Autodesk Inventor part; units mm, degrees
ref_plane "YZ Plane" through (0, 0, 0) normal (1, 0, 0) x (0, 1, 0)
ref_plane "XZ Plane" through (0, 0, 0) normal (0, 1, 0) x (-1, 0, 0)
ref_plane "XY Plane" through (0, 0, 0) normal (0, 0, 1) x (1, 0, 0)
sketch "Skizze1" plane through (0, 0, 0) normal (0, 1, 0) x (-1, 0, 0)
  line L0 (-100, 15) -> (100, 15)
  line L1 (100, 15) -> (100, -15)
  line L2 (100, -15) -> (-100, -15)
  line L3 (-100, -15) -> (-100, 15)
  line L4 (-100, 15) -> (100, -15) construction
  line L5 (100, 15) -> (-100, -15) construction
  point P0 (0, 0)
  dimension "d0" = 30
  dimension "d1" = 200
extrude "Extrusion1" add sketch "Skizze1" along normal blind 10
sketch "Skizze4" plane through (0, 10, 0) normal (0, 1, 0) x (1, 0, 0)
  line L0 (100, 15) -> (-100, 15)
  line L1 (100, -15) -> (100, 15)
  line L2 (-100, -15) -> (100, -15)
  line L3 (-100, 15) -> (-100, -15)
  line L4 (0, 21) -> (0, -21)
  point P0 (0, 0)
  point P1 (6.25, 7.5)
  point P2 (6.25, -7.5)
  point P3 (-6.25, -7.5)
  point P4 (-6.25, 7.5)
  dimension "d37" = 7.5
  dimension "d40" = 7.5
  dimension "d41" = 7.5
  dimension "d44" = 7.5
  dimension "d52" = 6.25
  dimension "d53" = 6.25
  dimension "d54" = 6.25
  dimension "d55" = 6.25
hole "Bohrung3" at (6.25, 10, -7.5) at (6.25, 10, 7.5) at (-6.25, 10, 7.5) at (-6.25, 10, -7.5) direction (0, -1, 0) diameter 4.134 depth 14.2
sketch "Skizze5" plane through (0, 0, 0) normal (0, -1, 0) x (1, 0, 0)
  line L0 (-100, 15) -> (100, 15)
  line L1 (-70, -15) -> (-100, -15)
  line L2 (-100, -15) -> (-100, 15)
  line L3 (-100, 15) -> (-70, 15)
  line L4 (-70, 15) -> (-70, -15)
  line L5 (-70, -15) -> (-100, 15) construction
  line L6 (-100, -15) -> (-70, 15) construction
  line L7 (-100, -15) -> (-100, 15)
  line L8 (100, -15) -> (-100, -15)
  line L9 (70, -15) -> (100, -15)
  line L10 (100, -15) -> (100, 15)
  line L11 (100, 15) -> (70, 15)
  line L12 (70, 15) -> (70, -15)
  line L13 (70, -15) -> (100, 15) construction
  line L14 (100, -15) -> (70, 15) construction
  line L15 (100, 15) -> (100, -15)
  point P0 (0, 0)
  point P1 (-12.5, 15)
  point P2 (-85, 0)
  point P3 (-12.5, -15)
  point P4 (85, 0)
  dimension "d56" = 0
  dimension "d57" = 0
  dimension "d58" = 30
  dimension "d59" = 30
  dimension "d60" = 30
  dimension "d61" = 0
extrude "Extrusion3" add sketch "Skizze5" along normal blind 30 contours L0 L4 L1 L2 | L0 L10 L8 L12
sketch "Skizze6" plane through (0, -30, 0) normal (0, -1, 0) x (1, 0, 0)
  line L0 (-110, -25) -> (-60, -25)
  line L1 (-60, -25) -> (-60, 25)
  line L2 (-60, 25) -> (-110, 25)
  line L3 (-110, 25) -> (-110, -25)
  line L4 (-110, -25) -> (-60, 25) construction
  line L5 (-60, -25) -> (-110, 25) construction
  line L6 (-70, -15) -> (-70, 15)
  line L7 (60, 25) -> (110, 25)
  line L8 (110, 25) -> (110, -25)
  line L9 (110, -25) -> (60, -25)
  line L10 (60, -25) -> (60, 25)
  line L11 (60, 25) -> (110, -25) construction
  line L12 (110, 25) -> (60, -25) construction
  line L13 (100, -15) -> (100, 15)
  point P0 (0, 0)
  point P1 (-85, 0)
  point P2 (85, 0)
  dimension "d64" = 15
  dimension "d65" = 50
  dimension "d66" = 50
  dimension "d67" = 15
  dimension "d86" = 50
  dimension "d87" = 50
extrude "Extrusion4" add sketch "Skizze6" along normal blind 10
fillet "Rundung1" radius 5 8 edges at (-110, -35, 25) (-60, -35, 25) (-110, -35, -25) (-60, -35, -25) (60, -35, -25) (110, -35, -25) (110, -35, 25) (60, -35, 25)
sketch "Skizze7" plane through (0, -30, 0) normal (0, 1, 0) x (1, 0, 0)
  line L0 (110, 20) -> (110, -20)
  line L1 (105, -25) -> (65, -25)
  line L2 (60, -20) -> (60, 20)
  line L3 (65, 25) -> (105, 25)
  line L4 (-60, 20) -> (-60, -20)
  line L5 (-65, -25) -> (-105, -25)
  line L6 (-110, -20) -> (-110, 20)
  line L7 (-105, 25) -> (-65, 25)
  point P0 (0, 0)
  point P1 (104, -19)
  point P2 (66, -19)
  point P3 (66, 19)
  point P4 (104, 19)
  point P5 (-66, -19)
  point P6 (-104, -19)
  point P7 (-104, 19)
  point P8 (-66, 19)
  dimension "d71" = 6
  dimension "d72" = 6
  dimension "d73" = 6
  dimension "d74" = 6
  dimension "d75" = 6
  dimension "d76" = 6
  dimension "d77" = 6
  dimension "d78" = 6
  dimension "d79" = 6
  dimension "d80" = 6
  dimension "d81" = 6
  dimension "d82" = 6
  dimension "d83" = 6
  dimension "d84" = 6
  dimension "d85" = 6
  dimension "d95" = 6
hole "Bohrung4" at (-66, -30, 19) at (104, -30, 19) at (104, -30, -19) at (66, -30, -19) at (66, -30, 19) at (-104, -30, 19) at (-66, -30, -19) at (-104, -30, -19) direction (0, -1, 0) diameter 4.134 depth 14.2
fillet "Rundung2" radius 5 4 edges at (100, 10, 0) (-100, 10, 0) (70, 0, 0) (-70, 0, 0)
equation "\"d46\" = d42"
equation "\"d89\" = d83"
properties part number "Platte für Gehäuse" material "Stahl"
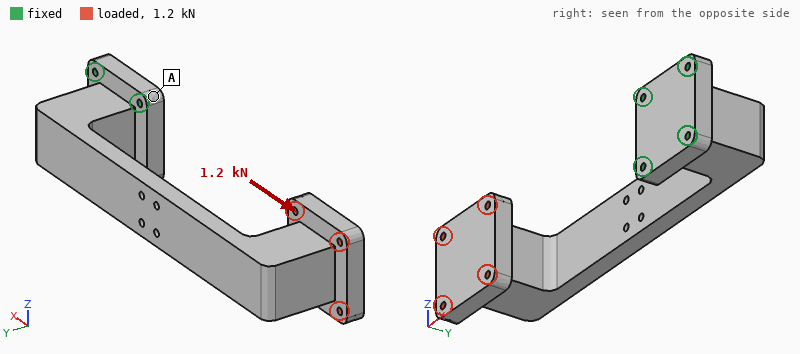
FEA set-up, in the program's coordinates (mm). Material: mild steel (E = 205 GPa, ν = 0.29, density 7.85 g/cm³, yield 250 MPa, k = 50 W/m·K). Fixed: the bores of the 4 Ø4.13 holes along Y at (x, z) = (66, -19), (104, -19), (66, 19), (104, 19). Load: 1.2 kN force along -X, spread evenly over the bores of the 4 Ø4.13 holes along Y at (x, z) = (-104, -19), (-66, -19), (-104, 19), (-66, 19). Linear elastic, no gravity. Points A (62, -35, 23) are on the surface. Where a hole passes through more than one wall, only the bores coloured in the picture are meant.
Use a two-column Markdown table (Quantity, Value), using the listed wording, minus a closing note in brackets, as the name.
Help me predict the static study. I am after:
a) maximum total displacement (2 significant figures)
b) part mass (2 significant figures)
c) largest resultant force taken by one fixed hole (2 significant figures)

| Quantity | Value |
|---|---|
| maximum total displacement | 1.7 mm |
| part mass | 1.3 kg |
| largest resultant force taken by one fixed hole | 320 N |
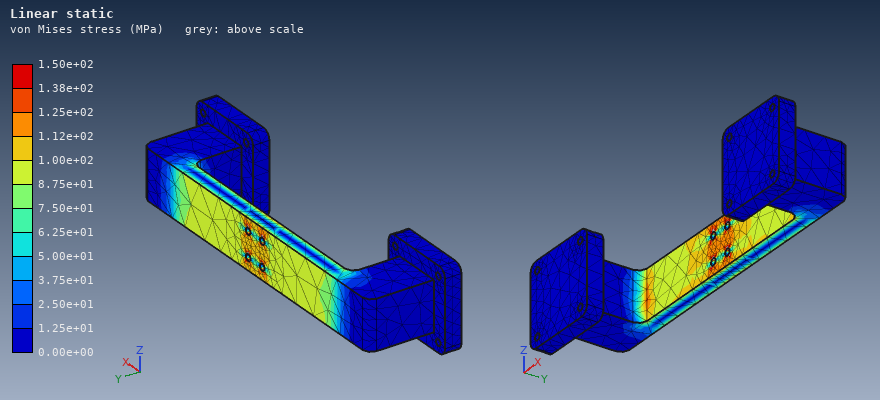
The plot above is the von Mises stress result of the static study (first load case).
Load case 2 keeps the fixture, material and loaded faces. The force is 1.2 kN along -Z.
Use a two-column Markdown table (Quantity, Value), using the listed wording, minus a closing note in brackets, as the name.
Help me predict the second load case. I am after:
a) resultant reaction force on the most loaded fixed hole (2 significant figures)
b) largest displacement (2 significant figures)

| Quantity | Value |
|---|---|
| resultant reaction force on the most loaded fixed hole | 2.1 kN |
| largest displacement | 1.2 mm |
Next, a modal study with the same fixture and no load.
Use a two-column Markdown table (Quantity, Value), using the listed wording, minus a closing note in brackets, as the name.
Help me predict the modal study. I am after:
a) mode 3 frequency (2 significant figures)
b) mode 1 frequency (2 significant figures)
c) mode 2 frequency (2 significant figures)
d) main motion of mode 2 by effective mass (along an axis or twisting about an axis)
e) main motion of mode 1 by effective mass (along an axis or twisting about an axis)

| Quantity | Value |
|---|---|
| mode 3 frequency | 790 Hz |
| mode 1 frequency | 130 Hz |
| mode 2 frequency | 280 Hz |
| main motion of mode 2 by effective mass | along Z |
| main motion of mode 1 by effective mass | along Y |
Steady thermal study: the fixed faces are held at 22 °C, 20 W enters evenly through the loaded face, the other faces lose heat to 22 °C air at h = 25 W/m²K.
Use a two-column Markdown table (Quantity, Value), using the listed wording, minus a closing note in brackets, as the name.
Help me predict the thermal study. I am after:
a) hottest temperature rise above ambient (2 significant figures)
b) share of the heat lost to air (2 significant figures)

| Quantity | Value |
|---|---|
| hottest temperature rise above ambient | 55 K |
| share of the heat lost to air | 91 % |
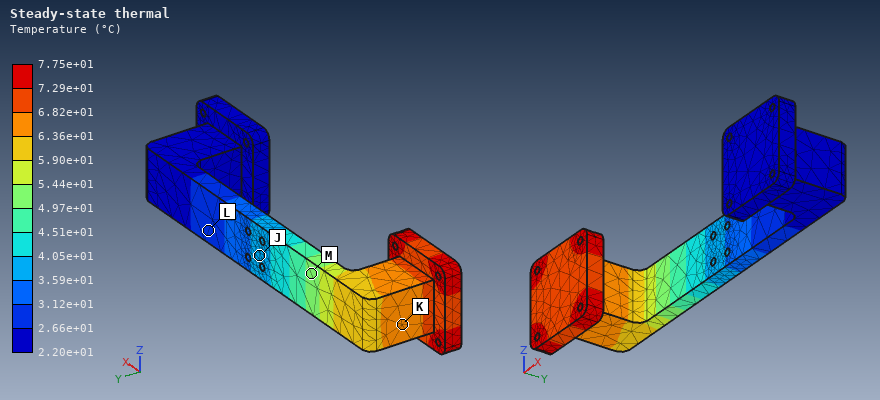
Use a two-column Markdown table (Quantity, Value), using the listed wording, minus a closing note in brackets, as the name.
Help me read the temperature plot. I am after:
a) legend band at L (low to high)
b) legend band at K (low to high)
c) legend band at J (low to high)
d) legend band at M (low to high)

| Quantity | Value |
|---|---|
| legend band at L | 2.66e+01 to 3.12e+01 °C |
| legend band at K | 6.36e+01 to 6.82e+01 °C |
| legend band at J | 3.59e+01 to 4.05e+01 °C |
| legend band at M | 4.97e+01 to 5.44e+01 °C |
